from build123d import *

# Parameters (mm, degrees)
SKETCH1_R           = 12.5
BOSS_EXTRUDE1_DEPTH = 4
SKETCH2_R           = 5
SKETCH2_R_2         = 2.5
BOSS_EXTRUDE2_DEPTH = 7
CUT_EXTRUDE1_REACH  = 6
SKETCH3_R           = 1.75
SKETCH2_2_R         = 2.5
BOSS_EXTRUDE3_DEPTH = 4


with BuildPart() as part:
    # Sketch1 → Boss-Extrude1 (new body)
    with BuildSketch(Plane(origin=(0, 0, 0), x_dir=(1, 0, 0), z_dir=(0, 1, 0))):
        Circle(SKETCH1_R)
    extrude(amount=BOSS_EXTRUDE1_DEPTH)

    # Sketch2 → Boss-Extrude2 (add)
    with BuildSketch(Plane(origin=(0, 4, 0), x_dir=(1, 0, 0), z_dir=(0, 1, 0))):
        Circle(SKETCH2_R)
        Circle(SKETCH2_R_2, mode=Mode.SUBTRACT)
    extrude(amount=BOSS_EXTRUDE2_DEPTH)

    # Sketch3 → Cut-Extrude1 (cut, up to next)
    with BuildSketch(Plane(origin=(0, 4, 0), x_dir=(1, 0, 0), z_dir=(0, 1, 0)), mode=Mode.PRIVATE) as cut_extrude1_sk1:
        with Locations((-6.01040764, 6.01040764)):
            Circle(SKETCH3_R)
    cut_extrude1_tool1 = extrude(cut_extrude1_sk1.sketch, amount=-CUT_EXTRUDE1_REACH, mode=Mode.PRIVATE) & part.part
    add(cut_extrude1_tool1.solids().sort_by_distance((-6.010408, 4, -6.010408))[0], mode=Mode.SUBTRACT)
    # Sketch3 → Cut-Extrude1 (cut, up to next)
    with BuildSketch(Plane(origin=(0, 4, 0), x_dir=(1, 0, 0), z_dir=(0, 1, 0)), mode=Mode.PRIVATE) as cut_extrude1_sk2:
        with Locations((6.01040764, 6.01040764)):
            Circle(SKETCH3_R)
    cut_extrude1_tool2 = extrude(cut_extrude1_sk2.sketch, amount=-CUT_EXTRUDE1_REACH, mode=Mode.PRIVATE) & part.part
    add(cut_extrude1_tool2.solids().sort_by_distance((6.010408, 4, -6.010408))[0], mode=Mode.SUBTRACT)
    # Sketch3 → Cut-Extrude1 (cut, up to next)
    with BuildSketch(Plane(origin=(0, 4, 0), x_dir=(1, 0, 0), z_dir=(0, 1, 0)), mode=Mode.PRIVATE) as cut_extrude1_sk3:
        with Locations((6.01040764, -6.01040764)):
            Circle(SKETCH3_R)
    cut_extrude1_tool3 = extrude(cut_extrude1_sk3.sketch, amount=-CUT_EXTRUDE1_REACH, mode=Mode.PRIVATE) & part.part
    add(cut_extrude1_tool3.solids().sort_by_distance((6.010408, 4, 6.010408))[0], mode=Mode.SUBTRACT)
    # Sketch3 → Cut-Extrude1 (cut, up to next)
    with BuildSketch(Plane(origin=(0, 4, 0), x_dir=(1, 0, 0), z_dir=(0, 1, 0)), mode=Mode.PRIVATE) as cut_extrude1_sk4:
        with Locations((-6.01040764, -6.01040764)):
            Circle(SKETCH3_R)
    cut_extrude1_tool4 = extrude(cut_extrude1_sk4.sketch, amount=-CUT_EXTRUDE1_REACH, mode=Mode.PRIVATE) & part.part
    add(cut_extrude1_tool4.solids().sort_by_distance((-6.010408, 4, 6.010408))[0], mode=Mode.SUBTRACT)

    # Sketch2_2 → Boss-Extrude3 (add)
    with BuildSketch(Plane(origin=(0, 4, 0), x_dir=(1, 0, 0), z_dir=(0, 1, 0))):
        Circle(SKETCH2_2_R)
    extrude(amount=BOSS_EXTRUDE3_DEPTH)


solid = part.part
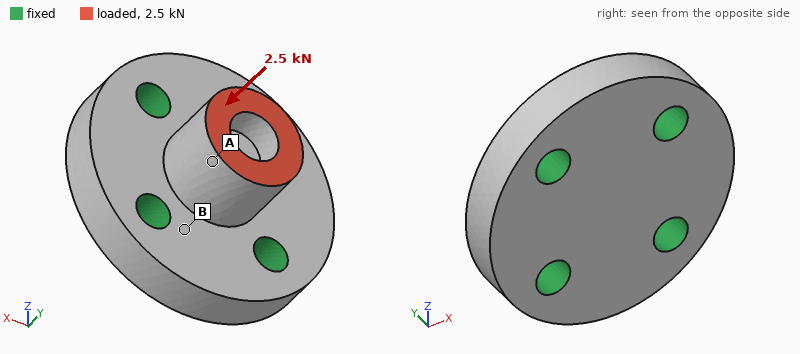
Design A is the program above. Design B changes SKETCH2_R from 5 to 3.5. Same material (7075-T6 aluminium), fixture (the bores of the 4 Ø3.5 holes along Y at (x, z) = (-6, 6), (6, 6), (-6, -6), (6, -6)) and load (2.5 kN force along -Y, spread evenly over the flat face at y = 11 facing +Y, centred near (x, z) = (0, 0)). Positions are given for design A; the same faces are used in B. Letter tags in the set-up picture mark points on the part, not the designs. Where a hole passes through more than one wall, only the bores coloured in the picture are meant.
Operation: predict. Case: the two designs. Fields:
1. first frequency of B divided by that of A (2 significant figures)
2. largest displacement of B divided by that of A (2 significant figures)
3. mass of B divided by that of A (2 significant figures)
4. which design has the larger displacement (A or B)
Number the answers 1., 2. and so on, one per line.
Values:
1. 1.0
2. 2.2
3. 0.88
4. B
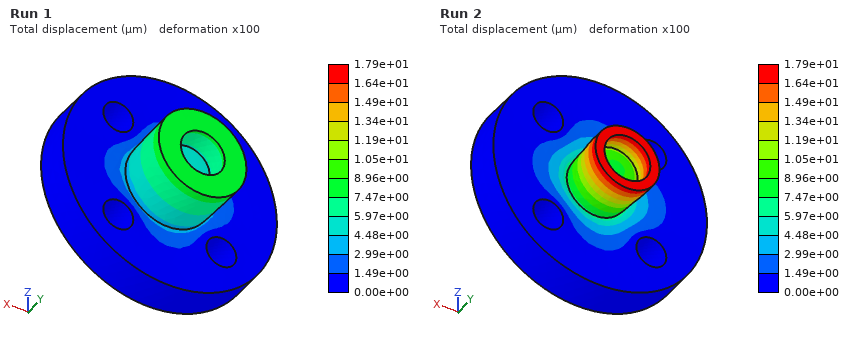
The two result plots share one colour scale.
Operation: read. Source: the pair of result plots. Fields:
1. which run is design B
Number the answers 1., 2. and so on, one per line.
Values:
1. Run 2
